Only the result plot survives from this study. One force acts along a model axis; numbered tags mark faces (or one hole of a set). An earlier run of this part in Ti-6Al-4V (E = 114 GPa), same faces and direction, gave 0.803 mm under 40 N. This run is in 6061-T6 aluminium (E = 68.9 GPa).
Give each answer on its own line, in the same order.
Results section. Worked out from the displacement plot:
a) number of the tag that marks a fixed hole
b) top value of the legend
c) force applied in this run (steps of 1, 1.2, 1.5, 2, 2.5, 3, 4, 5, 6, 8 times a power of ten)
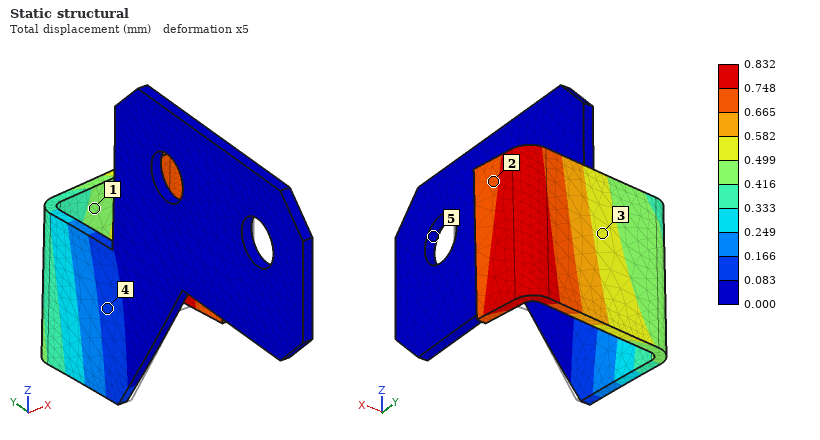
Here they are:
5
0.832 mm
25 N
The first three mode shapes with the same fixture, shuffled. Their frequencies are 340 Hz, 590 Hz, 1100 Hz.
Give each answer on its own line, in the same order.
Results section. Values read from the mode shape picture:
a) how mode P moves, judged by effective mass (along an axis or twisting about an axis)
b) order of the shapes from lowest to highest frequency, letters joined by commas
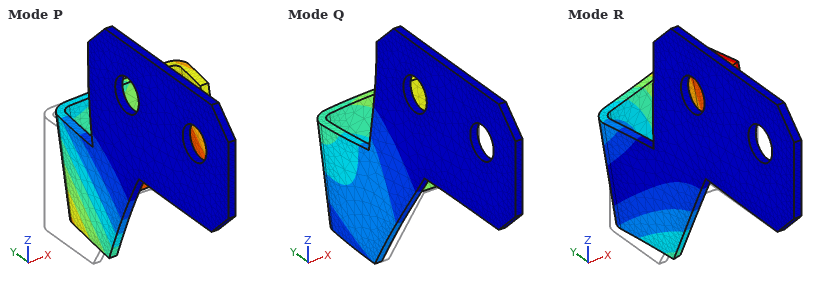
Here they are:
along X
P, R, Q
